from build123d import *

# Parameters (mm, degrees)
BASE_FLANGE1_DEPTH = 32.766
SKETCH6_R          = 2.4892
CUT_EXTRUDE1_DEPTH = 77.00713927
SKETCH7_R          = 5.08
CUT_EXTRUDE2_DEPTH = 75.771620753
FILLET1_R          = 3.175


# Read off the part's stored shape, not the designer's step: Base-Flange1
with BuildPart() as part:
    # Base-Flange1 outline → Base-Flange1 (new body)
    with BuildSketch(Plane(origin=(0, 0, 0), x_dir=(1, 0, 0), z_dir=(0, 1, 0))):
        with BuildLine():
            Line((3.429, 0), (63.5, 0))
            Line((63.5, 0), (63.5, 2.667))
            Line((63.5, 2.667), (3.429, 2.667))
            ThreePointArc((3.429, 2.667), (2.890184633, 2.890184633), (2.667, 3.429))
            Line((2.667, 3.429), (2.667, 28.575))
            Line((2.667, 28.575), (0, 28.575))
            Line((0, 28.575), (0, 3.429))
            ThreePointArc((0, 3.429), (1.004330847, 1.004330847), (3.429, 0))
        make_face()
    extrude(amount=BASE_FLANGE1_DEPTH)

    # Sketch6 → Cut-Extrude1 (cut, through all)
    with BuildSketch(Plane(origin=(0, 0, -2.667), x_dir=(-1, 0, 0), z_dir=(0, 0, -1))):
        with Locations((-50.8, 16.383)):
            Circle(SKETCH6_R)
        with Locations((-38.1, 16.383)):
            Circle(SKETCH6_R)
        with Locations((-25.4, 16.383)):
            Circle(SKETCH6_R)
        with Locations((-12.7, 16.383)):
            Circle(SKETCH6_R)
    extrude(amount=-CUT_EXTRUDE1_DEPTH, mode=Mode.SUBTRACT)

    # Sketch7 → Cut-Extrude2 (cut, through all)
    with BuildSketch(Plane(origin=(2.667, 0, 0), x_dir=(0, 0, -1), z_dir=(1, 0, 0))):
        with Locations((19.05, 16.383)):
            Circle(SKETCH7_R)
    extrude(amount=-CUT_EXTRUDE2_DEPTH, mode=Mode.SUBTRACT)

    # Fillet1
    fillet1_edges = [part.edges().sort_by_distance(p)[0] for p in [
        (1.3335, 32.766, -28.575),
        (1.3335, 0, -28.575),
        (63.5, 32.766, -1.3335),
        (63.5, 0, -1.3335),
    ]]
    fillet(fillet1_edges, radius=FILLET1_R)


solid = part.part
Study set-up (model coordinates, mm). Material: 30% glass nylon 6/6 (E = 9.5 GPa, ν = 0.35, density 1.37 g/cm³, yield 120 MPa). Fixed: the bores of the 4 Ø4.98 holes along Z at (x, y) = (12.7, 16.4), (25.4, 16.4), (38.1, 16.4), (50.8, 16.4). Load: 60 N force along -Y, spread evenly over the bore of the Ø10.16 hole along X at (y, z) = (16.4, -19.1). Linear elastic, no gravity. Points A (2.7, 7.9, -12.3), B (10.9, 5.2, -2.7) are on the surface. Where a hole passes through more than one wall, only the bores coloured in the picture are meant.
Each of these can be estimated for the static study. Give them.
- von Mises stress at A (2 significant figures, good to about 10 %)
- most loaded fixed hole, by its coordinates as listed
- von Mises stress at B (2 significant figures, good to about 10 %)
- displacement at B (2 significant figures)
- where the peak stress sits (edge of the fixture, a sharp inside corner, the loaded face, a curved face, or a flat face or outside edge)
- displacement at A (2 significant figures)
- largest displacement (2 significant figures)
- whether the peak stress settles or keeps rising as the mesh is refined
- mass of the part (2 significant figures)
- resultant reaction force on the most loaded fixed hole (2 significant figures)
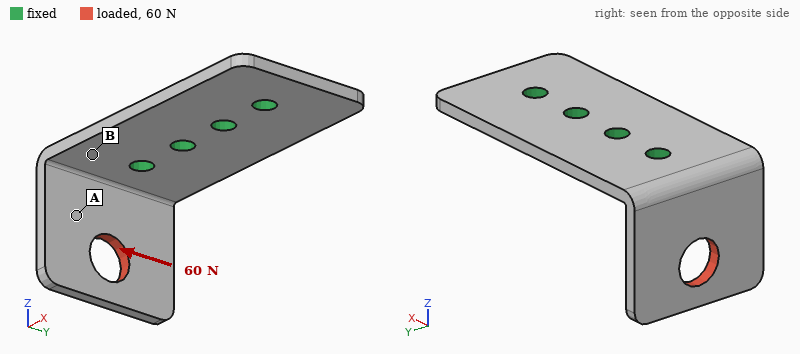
4.4 MPa
(12.7, 16.4)
10 MPa
0.066 mm
edge of the fixture
0.18 mm
0.40 mm
keeps rising
10.0 g
77 N
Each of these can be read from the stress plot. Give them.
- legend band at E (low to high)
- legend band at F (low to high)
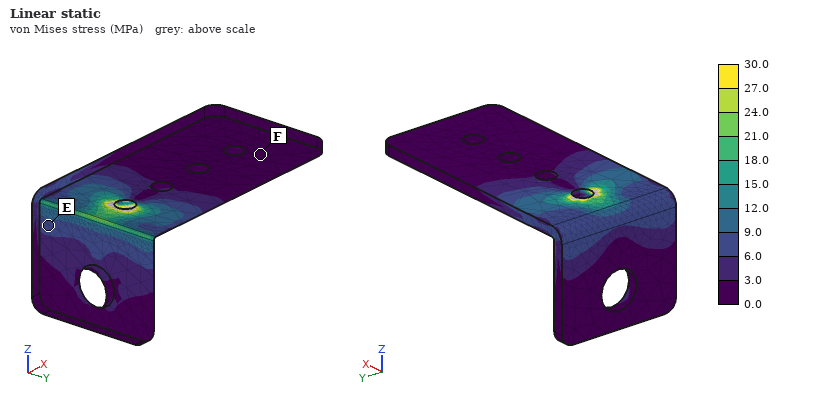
6.0 to 9.0 MPa
0.0 to 3.0 MPa
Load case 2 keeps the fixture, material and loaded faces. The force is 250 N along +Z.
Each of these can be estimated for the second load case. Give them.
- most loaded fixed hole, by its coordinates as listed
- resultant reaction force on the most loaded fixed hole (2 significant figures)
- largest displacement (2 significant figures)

(12.7, 16.4)
310 N
0.91 mm
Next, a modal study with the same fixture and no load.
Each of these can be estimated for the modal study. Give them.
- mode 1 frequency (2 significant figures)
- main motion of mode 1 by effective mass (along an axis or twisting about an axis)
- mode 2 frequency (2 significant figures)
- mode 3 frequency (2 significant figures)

1000 Hz
along X
1400 Hz
2800 Hz
